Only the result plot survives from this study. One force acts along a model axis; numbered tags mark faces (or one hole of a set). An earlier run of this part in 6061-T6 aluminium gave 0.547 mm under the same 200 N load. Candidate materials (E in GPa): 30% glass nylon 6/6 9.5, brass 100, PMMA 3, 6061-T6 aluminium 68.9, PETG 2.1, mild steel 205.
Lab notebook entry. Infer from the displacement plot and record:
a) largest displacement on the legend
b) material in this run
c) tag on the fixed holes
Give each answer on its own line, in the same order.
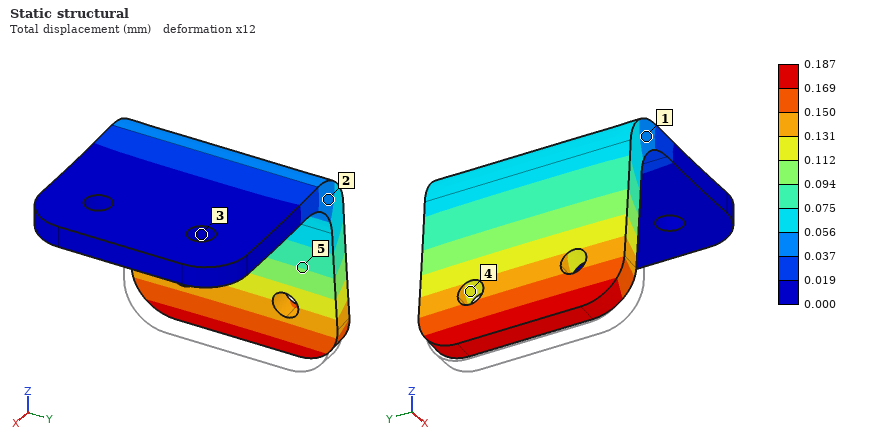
0.187 mm
mild steel
3
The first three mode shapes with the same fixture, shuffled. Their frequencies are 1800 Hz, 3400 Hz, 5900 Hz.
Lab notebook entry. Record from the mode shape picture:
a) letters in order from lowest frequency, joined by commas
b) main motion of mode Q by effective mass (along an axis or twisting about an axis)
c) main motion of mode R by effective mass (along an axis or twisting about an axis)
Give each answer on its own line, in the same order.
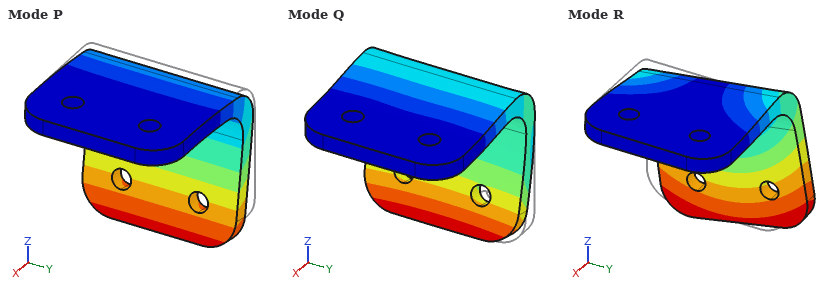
P, R, Q
along Z
along Y
